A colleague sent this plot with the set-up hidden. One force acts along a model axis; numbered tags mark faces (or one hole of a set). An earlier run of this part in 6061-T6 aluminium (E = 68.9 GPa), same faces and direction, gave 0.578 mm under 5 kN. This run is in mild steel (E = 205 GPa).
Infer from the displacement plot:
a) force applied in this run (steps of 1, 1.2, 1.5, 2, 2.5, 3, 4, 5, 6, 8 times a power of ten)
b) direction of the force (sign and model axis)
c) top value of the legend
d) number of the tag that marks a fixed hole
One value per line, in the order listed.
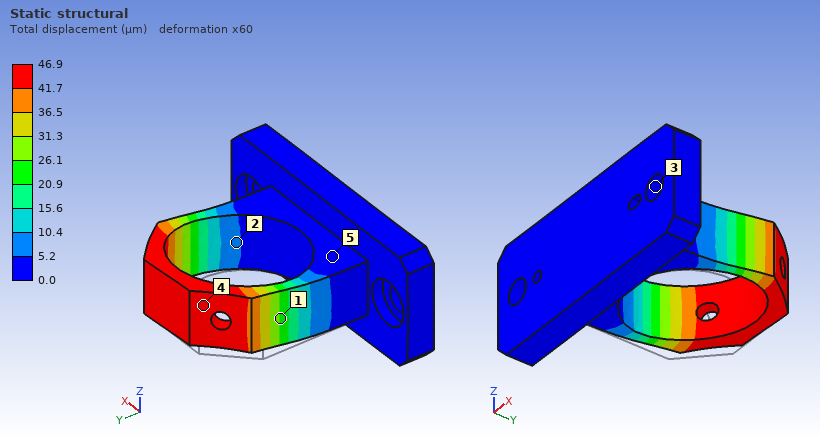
1.2 kN
+X
46.9 µm
3
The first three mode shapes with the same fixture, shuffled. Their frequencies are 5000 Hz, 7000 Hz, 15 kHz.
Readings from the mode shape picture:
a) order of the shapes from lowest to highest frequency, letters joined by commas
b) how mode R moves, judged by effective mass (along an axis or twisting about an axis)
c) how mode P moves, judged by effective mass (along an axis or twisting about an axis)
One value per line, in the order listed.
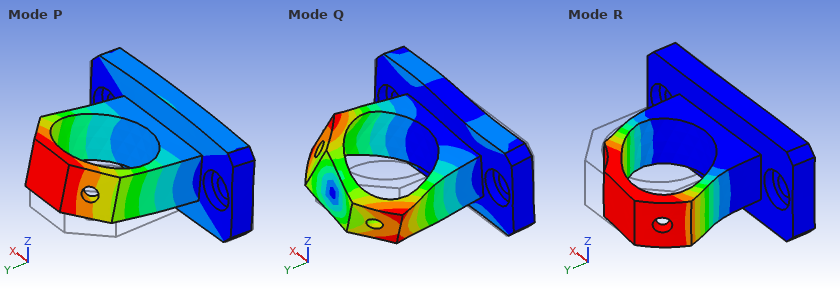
P, R, Q
along X
along Z
